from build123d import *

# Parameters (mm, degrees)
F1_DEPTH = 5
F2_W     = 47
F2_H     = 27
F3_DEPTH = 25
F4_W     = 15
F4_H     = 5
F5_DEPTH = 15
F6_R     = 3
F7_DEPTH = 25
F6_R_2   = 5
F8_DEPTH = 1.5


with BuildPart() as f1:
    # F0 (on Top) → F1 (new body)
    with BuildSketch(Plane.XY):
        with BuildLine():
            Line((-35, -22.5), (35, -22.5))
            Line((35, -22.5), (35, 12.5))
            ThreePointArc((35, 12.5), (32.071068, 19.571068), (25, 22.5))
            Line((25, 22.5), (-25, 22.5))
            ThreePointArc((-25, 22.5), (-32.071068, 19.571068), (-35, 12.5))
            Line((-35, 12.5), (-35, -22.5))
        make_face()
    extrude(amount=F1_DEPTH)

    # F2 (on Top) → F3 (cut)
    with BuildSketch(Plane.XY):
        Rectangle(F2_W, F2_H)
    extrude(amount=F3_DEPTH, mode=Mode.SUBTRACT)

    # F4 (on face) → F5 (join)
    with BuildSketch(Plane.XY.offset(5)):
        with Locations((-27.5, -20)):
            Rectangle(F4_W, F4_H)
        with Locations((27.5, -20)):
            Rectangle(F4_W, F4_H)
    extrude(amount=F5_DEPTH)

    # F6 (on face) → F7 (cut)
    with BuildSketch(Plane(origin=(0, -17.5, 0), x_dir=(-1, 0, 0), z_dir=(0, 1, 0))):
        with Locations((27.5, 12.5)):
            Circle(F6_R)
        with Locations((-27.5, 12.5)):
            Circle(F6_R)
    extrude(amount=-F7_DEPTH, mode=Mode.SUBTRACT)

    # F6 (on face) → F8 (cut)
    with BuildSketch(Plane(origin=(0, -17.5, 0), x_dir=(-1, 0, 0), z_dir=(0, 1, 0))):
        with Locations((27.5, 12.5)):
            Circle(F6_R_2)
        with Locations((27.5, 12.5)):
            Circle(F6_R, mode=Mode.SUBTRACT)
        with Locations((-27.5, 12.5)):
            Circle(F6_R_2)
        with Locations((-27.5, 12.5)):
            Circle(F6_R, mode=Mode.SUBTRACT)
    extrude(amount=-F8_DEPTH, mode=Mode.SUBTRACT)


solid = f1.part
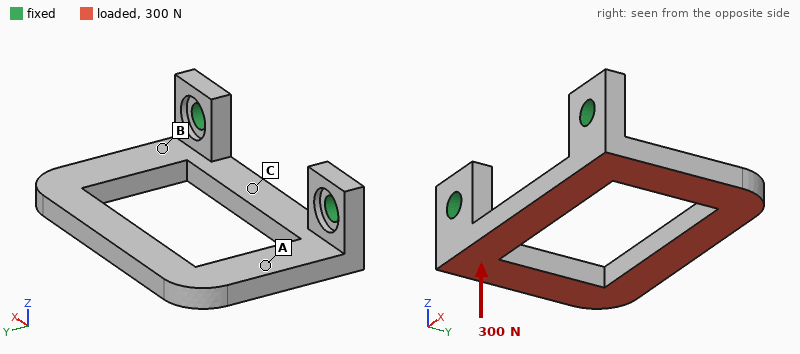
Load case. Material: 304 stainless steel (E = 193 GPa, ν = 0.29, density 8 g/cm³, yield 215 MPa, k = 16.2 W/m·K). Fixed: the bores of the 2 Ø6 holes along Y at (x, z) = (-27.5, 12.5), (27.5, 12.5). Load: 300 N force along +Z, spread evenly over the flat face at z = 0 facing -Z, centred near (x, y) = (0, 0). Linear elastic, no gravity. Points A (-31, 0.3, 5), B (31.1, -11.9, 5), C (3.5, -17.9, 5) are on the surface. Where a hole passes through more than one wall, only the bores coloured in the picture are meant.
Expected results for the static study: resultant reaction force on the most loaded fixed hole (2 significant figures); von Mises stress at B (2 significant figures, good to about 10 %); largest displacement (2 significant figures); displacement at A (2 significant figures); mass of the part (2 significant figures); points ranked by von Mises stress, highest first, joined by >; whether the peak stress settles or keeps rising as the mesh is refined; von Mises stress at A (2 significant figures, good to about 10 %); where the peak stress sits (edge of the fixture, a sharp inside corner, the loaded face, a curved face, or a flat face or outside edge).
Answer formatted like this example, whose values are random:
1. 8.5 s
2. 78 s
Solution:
1. 150 N
2. 39 MPa
3. 0.11 mm
4. 0.038 mm
5. 88 g
6. B > A > C
7. keeps rising
8. 21 MPa
9. edge of the fixture
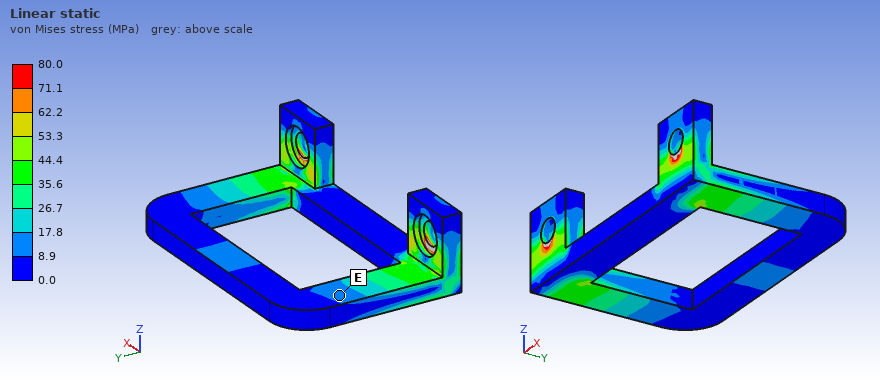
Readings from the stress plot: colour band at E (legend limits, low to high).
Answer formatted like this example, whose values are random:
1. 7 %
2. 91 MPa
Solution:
1. 8.9 to 17.8 MPa
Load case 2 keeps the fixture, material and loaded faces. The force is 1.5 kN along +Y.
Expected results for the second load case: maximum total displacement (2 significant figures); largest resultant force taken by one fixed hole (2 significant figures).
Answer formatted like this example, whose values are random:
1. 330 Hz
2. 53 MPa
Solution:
1. 0.14 mm
2. 750 N
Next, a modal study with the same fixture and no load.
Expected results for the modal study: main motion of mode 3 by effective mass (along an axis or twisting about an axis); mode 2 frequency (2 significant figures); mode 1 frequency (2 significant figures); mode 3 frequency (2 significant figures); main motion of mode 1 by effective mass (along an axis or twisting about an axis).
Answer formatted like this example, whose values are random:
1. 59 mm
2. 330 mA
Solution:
1. along X
2. 2400 Hz
3. 1200 Hz
4. 3500 Hz
5. along Z
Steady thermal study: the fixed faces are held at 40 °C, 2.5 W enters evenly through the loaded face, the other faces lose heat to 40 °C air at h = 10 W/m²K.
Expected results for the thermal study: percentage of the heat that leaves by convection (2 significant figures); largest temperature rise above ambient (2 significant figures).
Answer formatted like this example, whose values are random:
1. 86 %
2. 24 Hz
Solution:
1. 25 %
2. 26 K
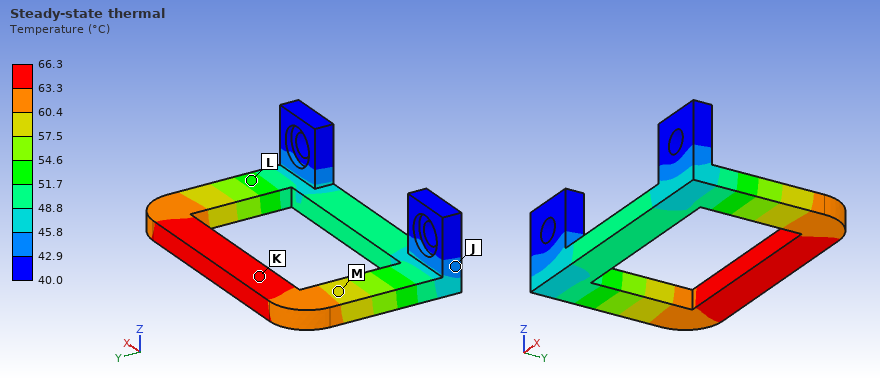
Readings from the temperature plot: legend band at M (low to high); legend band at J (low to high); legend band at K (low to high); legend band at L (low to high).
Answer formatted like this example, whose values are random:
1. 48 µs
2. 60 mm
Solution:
1. 57.5 to 60.4 °C
2. 42.9 to 45.8 °C
3. 63.3 to 66.3 °C
4. 51.7 to 54.6 °C
